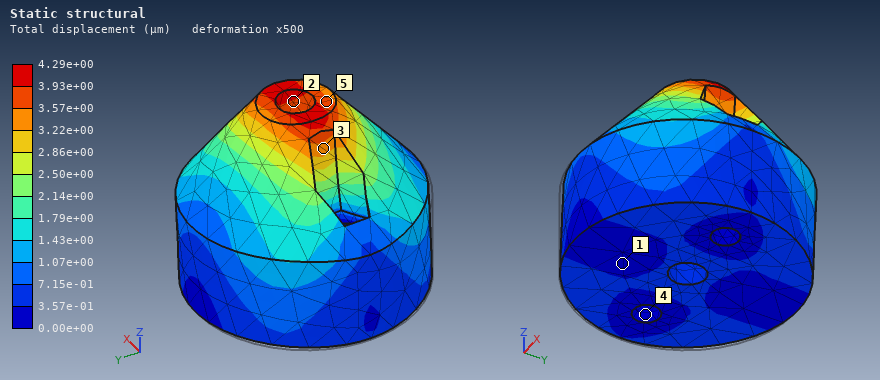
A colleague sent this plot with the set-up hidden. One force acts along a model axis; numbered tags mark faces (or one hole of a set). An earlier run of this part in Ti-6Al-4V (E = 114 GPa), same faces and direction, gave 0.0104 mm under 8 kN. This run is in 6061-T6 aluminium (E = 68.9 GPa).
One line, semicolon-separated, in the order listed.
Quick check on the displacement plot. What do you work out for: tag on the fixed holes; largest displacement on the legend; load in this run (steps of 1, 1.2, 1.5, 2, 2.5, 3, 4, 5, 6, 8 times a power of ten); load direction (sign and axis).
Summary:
4; 4.29e+00 µm; 2 kN; +X
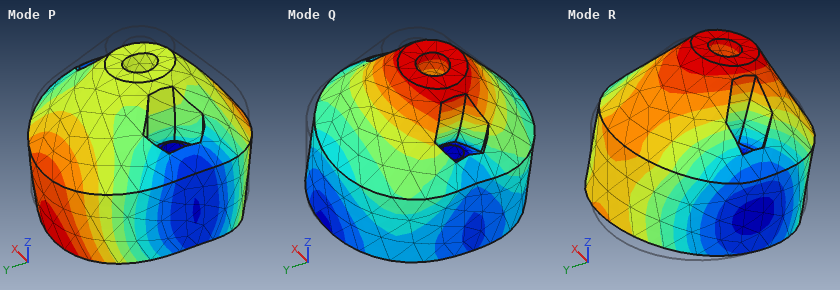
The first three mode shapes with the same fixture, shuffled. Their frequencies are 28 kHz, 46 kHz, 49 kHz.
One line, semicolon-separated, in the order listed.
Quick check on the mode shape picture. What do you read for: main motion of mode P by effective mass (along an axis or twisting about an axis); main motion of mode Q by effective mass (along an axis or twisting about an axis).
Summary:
along Z; along X
